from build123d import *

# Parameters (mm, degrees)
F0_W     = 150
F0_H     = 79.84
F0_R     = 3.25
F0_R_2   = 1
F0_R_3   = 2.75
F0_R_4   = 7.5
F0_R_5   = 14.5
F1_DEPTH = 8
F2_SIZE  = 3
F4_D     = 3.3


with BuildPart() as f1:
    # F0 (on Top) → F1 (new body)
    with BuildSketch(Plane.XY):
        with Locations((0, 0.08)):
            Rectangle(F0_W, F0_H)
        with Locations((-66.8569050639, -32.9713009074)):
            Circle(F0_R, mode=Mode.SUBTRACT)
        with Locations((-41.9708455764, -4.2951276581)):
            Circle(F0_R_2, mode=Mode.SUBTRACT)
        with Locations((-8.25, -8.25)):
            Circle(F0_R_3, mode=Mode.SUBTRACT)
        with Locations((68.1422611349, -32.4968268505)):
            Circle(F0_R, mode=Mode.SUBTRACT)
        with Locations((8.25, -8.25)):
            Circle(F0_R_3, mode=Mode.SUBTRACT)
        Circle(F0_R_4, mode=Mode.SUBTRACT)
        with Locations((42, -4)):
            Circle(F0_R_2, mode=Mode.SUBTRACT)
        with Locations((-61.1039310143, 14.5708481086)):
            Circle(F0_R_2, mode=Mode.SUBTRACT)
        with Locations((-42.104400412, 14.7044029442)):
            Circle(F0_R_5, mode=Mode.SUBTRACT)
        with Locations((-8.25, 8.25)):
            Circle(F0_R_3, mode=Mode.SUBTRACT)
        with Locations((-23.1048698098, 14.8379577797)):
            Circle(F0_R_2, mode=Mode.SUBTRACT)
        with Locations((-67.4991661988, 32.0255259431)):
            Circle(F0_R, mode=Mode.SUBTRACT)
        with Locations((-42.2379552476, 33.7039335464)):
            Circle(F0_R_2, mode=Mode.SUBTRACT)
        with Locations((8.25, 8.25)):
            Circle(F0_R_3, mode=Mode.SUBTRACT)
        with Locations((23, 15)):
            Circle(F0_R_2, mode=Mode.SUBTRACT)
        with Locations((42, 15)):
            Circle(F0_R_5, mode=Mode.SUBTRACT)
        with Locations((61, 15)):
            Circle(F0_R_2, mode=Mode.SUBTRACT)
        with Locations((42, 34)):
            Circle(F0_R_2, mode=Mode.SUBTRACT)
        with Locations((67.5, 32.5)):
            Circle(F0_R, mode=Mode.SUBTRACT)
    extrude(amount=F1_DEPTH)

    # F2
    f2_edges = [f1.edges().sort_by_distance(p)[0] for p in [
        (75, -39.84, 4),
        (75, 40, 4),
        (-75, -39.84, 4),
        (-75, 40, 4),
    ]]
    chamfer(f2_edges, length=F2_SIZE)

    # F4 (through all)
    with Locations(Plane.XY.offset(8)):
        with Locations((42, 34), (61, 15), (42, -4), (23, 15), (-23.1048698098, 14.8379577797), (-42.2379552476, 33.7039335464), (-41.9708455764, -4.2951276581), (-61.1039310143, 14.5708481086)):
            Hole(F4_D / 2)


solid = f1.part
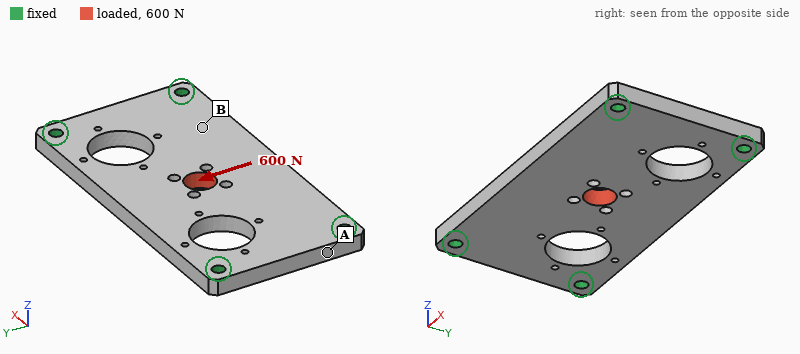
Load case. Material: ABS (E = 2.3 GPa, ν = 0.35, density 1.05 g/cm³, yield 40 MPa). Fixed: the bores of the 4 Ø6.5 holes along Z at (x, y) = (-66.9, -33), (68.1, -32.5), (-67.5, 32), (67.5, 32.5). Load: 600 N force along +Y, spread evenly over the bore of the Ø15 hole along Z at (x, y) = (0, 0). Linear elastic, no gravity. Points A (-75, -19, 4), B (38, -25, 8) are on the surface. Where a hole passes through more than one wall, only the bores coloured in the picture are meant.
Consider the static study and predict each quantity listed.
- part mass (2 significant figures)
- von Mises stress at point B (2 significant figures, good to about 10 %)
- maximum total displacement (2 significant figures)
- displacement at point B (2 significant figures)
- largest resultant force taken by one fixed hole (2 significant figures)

85 g
1.4 MPa
0.10 mm
0.050 mm
270 N
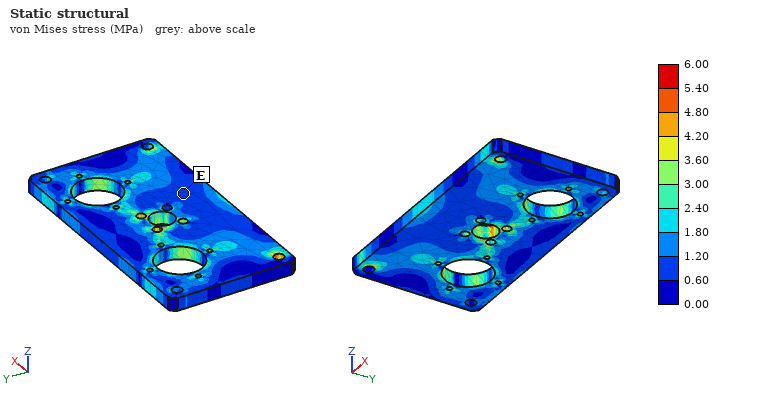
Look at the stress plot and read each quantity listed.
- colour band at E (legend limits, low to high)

0.60 to 1.20 MPa
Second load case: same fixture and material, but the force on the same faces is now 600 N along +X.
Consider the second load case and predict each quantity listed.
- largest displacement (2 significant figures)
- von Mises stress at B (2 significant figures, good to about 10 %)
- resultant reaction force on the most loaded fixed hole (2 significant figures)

47 µm
0.70 MPa
210 N
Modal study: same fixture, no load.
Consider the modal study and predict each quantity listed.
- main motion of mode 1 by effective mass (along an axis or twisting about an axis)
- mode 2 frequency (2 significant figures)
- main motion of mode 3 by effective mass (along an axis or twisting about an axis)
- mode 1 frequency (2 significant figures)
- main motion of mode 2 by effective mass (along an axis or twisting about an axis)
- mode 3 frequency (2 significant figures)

along Z
890 Hz
twisting about Y
570 Hz
twisting about X
1500 Hz
